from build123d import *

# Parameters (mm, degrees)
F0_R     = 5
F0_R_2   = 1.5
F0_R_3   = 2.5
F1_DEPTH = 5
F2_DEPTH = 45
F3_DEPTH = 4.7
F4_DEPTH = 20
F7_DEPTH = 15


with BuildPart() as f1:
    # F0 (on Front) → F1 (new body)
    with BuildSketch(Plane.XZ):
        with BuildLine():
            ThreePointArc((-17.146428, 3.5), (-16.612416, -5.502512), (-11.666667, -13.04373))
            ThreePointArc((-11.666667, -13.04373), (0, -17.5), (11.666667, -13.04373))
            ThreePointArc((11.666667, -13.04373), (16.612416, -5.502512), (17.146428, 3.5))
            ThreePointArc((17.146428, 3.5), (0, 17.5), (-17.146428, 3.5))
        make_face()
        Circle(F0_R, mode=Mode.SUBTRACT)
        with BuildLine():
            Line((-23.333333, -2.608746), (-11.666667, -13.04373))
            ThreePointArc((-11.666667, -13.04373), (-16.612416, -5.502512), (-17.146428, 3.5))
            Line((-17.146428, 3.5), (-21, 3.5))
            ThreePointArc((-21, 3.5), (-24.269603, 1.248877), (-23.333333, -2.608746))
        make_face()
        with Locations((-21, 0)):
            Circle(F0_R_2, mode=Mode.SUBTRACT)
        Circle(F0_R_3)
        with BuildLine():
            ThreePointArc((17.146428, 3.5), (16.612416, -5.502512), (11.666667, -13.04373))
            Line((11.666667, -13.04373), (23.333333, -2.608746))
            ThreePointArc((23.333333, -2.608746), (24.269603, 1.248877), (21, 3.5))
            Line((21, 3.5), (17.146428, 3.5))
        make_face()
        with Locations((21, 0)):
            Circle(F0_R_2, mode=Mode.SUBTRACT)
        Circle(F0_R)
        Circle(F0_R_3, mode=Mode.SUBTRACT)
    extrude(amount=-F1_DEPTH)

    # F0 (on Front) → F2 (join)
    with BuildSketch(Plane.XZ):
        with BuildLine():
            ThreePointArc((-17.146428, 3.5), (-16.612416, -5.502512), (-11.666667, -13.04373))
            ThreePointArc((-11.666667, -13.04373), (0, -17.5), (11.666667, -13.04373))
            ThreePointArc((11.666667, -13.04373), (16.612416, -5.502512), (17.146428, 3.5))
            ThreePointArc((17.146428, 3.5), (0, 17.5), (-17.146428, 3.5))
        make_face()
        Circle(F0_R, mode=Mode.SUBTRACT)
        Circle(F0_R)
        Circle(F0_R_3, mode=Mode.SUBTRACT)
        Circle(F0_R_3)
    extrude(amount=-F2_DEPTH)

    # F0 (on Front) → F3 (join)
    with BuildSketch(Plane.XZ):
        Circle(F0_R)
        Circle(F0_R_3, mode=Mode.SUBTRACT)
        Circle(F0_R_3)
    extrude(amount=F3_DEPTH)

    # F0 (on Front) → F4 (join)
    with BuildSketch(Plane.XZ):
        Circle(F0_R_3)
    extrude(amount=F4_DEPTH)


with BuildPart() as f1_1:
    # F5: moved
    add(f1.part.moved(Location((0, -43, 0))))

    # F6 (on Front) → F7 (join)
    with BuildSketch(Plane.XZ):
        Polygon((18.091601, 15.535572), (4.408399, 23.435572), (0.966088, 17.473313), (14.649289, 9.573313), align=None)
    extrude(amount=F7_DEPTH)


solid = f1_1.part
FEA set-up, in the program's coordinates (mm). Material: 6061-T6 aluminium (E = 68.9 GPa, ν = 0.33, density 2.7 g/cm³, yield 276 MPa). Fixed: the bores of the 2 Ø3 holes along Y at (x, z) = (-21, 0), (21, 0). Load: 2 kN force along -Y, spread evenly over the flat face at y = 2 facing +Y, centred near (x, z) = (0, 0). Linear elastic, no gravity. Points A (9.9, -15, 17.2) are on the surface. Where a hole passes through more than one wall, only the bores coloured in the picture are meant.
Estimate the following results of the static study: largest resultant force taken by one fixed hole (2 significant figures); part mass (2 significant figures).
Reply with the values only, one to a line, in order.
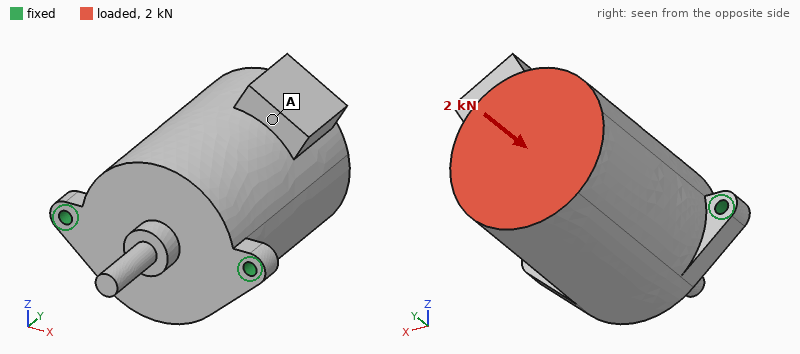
1.1 kN
120 g
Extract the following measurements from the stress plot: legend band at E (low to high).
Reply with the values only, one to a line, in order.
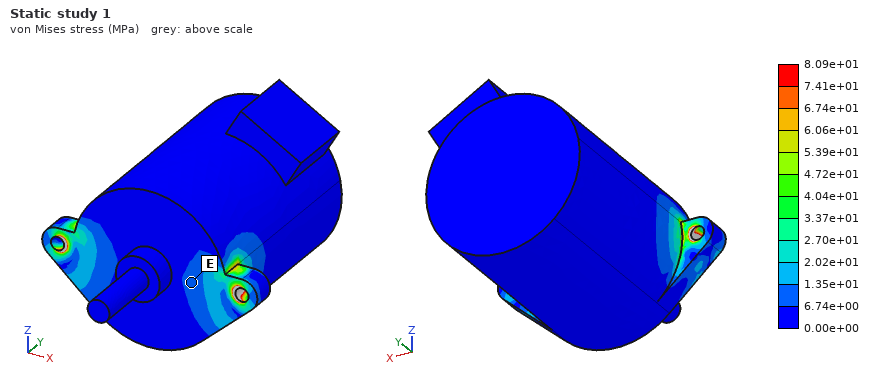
6.74e+00 to 1.35e+01 MPa
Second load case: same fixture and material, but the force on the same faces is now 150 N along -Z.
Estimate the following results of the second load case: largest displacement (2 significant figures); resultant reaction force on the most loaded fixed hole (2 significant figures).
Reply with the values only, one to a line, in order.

0.10 mm
83 N
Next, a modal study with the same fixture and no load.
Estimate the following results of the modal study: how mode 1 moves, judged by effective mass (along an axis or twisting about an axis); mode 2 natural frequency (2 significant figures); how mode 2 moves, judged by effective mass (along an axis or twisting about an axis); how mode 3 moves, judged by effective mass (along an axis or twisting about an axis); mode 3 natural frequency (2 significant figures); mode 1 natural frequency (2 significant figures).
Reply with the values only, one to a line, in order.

along Z
4900 Hz
along X
along Y
7000 Hz
960 Hz
